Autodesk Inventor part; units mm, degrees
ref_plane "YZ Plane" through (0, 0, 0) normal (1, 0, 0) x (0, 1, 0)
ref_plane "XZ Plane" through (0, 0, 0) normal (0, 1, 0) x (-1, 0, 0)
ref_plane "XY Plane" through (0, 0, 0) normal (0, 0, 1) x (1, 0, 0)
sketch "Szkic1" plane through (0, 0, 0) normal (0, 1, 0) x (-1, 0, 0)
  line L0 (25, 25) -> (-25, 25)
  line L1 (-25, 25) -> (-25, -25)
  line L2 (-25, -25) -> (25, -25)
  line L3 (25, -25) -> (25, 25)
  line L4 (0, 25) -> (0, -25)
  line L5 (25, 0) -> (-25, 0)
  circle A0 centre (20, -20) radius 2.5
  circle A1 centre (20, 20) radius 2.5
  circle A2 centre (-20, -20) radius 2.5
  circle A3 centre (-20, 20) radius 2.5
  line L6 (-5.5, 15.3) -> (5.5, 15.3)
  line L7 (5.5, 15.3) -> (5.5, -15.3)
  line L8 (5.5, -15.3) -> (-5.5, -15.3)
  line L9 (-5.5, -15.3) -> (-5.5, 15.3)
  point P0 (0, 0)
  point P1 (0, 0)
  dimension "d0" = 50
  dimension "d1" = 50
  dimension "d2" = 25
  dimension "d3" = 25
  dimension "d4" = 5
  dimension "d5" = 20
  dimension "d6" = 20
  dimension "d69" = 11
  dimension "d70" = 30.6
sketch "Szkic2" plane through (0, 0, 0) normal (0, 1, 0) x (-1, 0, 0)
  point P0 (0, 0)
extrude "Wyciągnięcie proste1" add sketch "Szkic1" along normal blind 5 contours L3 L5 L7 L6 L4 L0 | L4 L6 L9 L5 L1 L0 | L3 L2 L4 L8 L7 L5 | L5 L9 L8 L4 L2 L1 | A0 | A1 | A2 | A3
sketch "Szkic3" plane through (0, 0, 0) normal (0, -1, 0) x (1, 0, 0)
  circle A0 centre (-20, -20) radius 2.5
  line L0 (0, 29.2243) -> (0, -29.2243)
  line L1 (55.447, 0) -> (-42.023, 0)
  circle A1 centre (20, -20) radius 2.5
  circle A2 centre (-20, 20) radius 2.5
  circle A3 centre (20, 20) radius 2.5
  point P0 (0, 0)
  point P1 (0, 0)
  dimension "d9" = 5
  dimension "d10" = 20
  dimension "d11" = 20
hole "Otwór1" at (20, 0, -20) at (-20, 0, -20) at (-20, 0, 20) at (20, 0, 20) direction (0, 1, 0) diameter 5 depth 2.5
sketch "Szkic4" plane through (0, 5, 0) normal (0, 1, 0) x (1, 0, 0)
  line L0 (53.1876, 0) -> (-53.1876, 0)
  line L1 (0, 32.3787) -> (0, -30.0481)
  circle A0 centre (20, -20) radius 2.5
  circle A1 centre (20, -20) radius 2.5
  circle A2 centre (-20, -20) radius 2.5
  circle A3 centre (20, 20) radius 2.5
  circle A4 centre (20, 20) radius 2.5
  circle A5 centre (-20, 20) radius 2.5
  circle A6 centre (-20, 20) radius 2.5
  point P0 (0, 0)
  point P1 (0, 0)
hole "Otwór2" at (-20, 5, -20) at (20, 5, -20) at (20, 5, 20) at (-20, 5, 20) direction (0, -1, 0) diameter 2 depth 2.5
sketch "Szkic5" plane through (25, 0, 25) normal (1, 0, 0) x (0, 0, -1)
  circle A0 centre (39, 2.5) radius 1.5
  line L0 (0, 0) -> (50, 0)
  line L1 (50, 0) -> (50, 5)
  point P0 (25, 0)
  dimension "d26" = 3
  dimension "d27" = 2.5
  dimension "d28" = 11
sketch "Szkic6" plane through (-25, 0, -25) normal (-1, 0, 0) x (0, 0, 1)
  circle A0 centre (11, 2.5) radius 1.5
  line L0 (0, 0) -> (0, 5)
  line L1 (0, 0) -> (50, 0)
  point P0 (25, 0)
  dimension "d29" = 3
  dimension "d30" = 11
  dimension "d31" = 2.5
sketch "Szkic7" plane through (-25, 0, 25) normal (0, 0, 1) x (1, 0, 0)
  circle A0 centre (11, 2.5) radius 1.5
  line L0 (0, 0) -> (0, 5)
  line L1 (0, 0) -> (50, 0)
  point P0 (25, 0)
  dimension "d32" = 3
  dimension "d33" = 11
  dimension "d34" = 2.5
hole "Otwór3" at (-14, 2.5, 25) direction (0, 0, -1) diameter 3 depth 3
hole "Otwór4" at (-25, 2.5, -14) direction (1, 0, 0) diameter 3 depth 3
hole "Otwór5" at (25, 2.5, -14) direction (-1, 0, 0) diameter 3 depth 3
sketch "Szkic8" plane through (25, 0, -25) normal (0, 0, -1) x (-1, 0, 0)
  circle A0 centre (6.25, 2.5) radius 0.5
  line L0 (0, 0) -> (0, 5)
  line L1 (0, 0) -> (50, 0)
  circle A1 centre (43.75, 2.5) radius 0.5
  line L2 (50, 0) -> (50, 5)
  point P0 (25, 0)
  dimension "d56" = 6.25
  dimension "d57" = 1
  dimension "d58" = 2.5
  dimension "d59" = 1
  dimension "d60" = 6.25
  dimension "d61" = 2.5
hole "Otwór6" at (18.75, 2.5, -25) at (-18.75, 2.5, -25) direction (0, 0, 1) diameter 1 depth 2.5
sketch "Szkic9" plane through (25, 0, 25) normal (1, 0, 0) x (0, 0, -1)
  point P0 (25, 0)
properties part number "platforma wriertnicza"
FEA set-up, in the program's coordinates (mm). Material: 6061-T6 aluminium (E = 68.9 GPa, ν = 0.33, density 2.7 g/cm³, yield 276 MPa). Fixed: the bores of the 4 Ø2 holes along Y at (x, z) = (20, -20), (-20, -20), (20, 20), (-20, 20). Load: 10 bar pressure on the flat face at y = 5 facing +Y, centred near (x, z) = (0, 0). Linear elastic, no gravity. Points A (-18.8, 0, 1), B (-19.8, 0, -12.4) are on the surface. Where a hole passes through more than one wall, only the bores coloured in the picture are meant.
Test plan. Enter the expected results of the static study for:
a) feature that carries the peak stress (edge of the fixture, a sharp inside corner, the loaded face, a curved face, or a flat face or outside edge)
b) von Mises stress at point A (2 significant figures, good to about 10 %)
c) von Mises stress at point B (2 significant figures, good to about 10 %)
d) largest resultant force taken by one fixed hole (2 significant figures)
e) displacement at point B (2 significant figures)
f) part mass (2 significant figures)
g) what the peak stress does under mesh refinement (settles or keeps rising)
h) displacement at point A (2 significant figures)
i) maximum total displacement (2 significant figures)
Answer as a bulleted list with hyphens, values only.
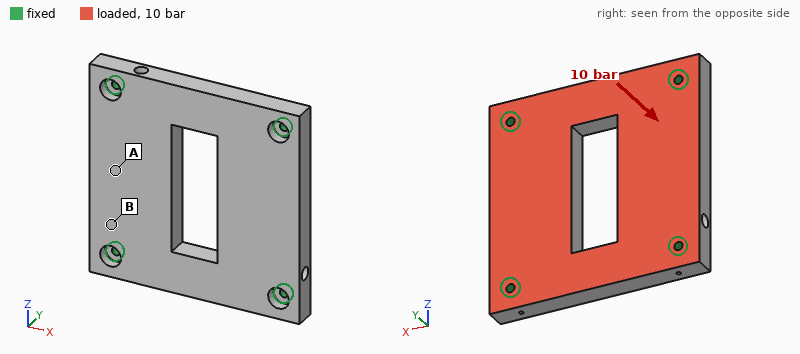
- edge of the fixture
- 31 MPa
- 19 MPa
- 690 N
- 17 µm
- 28 g
- keeps rising
- 29 µm
- 57 µm
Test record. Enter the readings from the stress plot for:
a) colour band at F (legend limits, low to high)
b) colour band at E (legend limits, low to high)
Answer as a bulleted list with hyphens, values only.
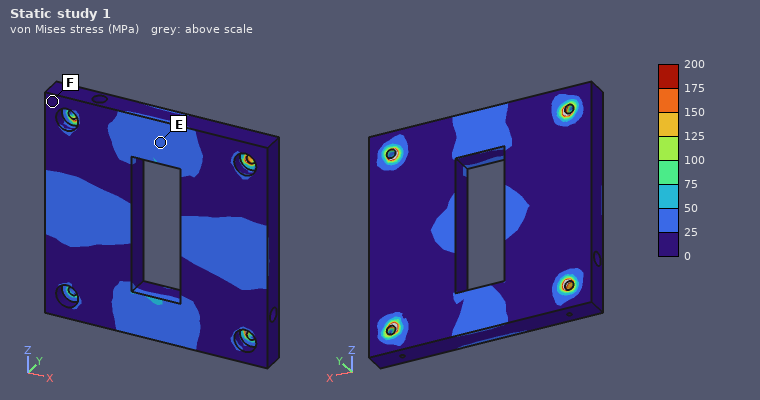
- 0 to 25 MPa
- 25 to 50 MPa
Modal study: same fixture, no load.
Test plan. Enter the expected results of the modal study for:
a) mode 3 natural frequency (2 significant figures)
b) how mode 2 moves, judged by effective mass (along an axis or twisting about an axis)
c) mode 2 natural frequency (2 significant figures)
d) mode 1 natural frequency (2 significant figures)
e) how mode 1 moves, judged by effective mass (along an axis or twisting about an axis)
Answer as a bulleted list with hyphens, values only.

- 11 kHz
- twisting about Z
- 11 kHz
- 7400 Hz
- along Y
